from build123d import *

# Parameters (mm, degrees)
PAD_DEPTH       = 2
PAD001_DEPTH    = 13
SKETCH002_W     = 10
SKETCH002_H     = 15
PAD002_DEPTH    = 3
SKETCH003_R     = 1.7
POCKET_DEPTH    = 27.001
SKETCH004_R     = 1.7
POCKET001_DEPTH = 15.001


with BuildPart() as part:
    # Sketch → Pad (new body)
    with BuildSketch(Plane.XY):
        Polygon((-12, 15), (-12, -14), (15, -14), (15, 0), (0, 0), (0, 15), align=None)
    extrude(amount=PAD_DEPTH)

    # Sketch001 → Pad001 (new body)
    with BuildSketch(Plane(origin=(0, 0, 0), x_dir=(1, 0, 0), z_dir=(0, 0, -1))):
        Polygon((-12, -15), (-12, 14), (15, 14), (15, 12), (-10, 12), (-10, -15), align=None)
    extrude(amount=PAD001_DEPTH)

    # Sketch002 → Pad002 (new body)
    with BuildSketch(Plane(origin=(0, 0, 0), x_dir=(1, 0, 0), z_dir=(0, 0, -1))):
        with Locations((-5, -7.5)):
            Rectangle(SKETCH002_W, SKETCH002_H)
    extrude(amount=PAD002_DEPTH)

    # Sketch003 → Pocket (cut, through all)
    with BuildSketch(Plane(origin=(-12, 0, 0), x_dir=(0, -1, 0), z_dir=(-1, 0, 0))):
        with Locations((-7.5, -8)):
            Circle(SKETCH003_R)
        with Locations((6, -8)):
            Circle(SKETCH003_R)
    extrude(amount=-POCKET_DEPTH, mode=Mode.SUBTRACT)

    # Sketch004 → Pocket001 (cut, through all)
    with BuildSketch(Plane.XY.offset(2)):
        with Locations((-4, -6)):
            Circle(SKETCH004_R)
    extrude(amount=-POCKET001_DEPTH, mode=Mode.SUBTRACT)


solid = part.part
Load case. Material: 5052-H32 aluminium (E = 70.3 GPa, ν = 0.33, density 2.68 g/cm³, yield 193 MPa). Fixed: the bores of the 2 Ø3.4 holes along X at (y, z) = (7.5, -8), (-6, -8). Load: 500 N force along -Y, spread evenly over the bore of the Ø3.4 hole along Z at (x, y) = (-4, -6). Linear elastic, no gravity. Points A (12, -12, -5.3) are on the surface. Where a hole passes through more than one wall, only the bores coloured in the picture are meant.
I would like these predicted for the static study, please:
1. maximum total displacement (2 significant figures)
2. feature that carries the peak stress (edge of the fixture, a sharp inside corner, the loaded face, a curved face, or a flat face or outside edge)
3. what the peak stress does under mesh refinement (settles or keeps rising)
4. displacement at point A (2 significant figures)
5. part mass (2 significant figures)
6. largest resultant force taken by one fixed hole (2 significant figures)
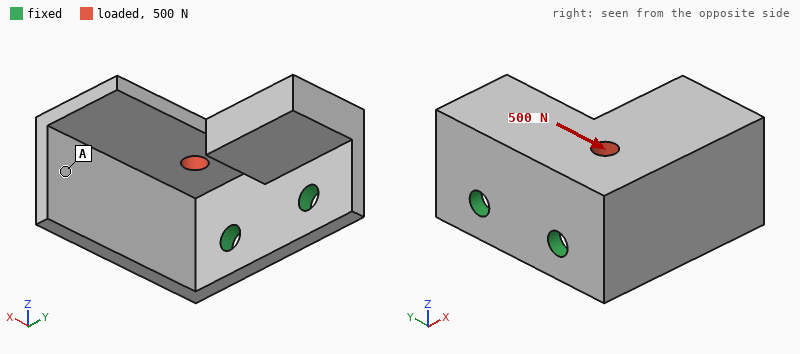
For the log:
84 µm
edge of the fixture
keeps rising
68 µm
7.8 g
420 N
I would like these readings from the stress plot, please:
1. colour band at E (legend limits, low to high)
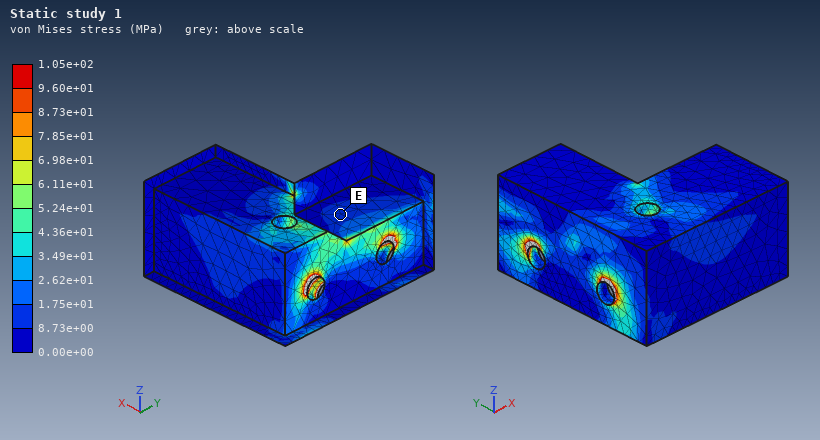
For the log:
8.73e+00 to 1.75e+01 MPa
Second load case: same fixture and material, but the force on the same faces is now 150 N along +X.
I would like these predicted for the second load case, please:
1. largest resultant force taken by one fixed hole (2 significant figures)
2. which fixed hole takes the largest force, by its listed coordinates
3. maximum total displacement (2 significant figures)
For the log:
130 N
(-6, -8)
78 µm
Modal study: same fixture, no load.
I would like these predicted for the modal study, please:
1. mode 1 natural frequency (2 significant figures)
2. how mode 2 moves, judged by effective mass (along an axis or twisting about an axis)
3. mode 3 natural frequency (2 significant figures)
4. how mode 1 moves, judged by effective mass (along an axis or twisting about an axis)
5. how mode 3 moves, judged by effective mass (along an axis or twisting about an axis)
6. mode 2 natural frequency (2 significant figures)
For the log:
2900 Hz
along Y
9200 Hz
along Z
along X
4300 Hz
